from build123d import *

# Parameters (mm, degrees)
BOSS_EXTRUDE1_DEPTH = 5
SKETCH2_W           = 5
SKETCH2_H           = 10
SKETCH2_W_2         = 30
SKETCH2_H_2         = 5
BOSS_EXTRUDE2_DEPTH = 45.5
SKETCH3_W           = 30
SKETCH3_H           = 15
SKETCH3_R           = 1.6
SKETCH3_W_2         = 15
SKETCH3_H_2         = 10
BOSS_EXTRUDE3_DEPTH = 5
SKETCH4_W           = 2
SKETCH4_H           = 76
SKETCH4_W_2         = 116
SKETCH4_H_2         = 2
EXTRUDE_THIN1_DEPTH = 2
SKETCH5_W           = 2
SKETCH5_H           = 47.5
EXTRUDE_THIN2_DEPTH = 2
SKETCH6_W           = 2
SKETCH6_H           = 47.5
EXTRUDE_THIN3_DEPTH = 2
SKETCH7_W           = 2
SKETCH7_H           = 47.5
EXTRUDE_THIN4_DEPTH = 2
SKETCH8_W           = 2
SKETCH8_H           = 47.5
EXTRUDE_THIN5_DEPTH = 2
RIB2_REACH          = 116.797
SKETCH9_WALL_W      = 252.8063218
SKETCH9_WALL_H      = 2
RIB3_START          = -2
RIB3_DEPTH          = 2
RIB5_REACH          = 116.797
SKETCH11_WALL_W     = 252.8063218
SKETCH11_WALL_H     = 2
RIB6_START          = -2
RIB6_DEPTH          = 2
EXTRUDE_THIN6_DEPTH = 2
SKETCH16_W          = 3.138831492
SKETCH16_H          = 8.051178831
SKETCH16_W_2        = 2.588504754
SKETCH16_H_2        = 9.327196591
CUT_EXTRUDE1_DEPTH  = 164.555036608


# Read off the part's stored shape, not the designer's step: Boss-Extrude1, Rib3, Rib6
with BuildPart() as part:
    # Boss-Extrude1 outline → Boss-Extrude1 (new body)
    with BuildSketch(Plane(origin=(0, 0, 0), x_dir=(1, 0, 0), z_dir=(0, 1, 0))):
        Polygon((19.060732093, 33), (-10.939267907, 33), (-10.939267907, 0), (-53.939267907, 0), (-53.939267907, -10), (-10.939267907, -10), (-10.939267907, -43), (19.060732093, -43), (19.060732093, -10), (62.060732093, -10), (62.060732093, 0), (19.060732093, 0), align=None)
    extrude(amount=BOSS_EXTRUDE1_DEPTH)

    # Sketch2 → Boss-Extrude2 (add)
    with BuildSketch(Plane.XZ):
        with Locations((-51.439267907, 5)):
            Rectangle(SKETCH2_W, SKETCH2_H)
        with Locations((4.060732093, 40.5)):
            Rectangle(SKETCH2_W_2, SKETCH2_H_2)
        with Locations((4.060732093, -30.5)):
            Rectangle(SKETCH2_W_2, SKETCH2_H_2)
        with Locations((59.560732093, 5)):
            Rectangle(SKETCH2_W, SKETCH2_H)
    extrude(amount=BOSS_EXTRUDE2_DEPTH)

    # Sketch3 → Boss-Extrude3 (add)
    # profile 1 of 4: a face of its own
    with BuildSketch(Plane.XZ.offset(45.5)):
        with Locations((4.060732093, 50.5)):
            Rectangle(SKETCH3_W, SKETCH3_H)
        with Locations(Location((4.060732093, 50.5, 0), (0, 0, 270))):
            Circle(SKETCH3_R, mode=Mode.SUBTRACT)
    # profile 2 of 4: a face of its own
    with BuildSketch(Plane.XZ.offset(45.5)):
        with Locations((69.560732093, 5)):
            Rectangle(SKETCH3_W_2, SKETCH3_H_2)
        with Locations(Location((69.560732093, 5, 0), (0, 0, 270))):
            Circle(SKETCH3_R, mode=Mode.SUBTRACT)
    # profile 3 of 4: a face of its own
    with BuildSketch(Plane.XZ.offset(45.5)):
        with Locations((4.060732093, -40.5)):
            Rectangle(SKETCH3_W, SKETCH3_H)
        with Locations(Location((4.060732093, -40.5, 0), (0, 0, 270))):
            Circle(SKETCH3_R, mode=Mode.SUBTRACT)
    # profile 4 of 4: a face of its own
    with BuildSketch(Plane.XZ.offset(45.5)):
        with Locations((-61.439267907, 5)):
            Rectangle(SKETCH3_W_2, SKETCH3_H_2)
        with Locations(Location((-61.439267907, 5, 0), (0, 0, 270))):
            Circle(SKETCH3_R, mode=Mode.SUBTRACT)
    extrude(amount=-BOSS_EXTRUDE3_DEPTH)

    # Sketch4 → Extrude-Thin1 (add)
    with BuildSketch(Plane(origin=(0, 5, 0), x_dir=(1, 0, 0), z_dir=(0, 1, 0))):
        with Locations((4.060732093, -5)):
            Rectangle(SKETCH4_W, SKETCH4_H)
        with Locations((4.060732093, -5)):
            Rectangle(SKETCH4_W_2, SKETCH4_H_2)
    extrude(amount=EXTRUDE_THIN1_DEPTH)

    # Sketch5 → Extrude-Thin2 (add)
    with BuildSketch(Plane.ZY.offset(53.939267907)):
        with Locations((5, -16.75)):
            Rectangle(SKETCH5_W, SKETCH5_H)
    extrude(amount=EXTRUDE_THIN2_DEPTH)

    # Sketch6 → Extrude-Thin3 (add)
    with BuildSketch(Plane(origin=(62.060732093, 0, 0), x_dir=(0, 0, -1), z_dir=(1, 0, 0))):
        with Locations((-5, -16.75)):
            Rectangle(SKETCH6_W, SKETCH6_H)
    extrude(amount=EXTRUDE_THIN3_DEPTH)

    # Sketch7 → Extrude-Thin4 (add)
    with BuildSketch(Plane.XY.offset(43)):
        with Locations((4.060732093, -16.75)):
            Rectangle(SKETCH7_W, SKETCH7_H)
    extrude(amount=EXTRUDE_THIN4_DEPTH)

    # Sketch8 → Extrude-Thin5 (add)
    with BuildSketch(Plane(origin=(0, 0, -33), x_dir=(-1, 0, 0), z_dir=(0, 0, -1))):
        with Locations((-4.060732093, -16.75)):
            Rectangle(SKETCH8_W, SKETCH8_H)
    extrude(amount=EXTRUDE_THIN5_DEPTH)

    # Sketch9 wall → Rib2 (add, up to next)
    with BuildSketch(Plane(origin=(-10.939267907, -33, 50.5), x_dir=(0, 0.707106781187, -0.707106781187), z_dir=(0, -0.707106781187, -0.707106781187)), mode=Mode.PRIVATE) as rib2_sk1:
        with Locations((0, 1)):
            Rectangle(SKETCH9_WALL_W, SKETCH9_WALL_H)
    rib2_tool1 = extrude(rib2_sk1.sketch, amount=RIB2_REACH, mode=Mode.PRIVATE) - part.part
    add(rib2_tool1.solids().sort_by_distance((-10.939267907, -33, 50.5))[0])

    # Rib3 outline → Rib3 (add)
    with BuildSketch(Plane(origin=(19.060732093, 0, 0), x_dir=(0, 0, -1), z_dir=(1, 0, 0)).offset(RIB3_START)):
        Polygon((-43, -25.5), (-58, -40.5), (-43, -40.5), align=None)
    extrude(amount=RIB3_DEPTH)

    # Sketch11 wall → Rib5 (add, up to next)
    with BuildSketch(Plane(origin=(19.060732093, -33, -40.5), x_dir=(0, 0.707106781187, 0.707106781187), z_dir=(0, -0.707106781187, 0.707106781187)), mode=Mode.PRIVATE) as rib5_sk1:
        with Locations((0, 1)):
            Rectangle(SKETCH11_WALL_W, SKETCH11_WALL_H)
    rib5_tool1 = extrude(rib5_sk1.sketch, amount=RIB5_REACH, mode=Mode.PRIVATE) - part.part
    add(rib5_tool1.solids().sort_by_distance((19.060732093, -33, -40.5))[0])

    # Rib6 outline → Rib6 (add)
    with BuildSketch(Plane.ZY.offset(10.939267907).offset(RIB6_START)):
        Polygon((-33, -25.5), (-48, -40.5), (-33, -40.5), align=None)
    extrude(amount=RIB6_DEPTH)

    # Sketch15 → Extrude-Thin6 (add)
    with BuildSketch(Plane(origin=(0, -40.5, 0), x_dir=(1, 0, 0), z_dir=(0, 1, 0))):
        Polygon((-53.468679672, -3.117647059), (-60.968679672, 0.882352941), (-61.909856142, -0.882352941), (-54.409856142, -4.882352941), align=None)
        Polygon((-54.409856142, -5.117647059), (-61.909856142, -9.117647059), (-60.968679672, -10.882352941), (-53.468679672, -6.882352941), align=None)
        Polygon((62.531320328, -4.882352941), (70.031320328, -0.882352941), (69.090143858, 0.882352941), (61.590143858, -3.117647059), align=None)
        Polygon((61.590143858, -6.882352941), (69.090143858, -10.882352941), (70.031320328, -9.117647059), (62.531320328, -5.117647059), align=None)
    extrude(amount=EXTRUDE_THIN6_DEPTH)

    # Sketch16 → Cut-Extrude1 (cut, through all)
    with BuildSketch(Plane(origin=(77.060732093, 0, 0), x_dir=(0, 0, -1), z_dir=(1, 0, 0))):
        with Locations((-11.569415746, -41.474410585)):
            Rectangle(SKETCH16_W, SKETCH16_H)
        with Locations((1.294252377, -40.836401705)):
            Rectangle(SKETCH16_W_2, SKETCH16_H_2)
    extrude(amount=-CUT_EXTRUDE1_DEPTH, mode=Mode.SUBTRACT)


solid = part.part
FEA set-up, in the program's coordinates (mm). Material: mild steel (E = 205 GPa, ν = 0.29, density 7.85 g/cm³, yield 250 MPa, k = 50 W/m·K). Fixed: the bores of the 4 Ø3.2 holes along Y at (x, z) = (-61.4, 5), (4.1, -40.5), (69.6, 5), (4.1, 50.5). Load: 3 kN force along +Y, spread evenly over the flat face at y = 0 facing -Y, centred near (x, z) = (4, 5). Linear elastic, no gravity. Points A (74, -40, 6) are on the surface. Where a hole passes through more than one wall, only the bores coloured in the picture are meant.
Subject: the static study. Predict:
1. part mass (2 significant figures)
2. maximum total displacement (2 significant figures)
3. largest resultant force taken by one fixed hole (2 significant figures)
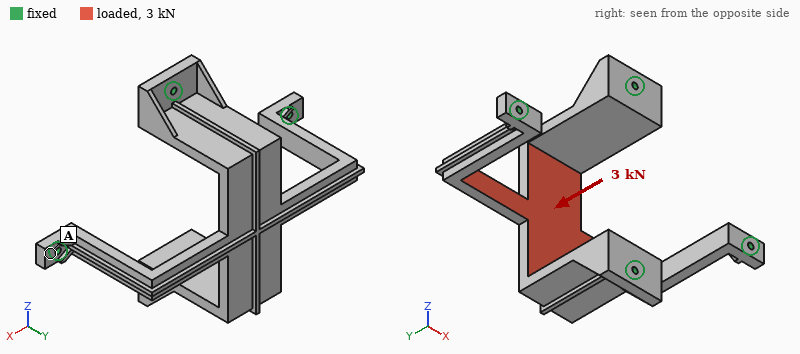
330 g
58 µm
1.2 kN
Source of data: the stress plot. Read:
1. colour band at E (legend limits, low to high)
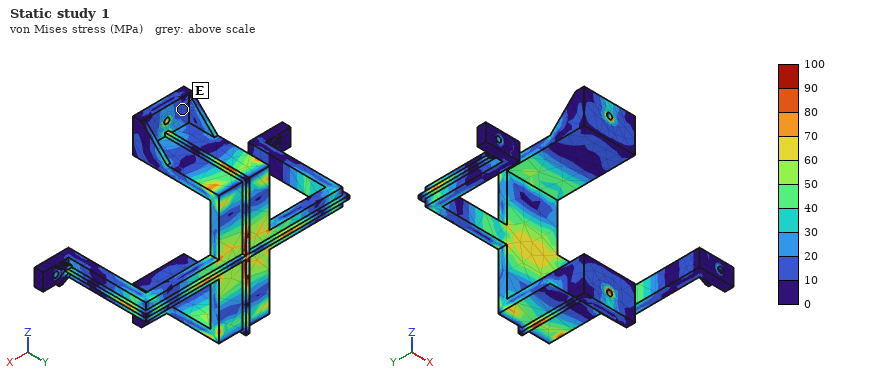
10 to 20 MPa
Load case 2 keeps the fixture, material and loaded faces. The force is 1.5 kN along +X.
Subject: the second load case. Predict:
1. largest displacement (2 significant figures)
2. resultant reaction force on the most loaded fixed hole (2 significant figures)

0.11 mm
530 N
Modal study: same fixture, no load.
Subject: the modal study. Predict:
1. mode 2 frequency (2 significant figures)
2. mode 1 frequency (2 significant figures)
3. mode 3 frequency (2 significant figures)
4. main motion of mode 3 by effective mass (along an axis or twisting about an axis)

1400 Hz
1400 Hz
2000 Hz
twisting about Y
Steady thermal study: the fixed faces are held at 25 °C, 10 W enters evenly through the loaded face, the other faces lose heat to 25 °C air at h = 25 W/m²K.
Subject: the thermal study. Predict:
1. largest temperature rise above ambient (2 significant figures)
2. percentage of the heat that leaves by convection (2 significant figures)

22 K
49 %
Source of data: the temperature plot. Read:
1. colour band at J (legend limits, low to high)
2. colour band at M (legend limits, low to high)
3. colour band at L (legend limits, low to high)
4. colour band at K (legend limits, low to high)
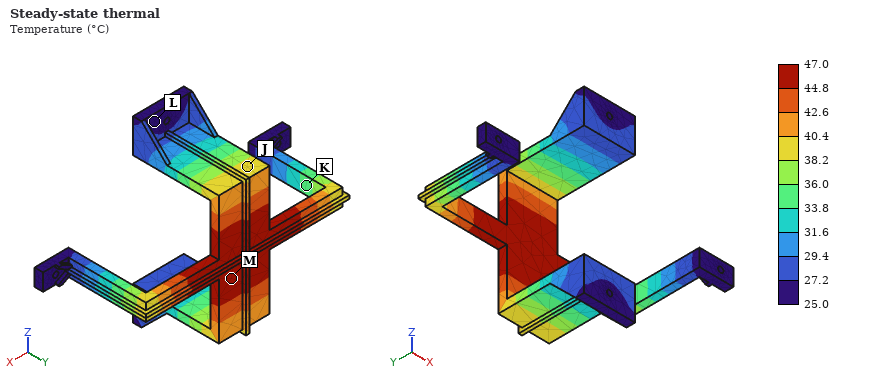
38.2 to 40.4 °C
44.8 to 47.0 °C
25.0 to 27.2 °C
33.8 to 36.0 °C
